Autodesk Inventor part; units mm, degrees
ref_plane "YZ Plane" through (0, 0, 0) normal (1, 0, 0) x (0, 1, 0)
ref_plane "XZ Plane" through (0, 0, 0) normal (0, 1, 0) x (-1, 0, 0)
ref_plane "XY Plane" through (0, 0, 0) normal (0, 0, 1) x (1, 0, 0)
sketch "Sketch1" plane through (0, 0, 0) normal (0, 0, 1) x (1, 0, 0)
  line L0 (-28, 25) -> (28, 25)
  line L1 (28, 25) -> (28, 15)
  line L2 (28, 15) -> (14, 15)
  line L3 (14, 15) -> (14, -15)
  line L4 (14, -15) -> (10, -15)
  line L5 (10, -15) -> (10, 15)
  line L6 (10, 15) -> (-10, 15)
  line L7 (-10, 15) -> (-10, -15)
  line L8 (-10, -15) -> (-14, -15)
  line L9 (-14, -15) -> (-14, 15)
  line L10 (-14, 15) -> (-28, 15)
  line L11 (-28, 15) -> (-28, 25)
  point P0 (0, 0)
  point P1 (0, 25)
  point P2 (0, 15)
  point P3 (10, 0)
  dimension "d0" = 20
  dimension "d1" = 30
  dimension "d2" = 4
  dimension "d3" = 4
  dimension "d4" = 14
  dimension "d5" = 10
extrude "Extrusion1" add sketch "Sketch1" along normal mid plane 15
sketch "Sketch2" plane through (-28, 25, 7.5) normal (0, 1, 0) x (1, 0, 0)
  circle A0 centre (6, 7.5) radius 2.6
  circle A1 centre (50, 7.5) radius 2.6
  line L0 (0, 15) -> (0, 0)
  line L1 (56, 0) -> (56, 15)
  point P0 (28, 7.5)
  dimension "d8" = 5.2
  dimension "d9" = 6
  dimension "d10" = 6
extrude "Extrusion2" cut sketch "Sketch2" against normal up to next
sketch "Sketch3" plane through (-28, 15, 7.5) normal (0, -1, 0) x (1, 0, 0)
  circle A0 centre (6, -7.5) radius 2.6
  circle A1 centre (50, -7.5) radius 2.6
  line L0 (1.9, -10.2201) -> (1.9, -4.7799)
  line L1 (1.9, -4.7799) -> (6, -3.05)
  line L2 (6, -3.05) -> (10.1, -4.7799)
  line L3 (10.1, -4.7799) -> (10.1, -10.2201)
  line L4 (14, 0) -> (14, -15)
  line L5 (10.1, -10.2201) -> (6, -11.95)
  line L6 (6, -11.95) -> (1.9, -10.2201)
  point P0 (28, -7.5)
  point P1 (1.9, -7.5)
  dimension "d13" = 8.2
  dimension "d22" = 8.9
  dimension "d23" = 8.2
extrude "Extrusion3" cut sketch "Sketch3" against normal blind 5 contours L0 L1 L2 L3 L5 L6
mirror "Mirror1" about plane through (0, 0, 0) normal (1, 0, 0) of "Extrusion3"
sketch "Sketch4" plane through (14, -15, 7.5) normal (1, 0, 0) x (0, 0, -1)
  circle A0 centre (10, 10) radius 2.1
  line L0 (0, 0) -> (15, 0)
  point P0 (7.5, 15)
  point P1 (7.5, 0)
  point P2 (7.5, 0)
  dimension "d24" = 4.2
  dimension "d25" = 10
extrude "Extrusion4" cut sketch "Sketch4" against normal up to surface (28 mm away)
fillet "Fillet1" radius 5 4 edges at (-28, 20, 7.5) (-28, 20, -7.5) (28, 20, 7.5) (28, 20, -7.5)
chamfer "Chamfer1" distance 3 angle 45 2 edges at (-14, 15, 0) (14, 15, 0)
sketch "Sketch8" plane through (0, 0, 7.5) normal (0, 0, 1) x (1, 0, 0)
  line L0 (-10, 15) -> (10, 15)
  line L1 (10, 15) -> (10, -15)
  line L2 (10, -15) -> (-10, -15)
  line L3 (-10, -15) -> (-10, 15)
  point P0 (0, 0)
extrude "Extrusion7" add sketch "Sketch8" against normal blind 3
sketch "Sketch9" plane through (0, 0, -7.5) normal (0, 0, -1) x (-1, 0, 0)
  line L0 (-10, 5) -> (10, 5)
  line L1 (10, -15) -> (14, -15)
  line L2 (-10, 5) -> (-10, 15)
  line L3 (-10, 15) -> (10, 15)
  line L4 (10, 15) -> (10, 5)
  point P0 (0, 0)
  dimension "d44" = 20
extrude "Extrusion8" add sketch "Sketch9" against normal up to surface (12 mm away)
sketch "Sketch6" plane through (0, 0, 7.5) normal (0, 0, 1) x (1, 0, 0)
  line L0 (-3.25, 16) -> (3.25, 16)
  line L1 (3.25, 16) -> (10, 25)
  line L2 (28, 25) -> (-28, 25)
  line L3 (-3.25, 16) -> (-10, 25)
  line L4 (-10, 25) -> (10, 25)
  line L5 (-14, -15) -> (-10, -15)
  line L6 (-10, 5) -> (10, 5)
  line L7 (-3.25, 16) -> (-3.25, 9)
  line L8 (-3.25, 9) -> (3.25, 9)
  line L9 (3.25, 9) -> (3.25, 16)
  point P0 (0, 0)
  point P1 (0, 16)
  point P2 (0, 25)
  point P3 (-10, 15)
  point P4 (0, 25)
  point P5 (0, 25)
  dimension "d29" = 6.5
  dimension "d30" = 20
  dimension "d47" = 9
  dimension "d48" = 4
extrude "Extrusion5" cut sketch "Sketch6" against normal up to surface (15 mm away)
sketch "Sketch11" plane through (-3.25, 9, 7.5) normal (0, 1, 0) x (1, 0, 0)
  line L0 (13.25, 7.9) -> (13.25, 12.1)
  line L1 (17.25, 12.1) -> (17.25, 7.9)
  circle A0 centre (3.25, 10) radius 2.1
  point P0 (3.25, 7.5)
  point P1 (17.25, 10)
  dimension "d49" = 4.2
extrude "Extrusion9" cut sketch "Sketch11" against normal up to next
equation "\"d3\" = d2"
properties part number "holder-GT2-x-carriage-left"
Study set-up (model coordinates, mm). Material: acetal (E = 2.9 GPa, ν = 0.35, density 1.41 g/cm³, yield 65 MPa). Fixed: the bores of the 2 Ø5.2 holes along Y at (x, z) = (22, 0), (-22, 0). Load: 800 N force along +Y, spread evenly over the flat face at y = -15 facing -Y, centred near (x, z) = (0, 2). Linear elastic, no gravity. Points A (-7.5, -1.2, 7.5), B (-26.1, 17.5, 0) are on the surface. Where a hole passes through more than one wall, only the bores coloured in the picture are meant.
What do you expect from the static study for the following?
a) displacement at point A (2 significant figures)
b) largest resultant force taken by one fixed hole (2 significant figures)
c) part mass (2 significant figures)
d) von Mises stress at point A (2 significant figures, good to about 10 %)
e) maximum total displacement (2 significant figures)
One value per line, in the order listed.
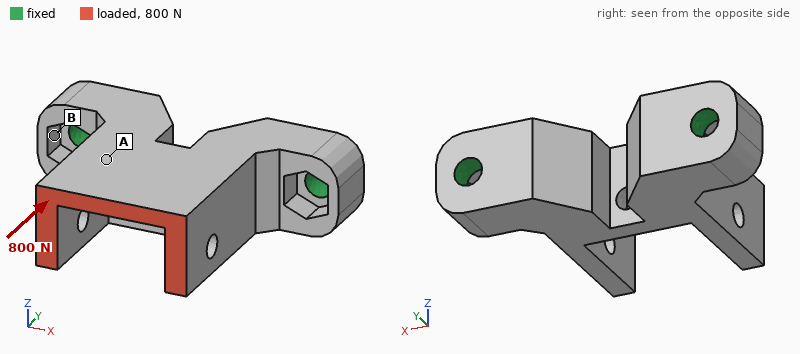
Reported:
0.16 mm
460 N
18 g
4.0 MPa
0.22 mm
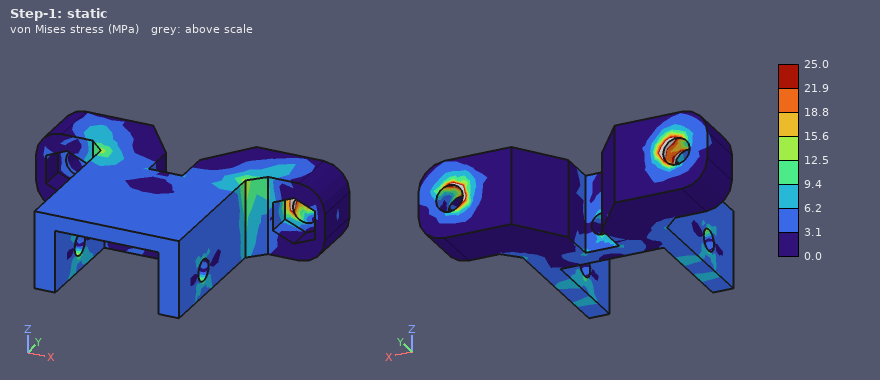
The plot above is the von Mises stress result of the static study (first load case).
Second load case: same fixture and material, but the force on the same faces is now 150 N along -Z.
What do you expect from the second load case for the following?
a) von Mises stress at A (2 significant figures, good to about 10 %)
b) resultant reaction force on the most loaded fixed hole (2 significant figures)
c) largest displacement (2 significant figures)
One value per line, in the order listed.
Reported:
3.9 MPa
79 N
0.82 mm
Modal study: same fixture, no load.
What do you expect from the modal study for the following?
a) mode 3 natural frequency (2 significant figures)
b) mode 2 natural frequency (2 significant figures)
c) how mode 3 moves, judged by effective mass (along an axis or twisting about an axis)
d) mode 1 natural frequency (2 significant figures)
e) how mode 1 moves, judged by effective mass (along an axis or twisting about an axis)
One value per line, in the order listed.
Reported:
3600 Hz
2400 Hz
along X
1300 Hz
along Z
